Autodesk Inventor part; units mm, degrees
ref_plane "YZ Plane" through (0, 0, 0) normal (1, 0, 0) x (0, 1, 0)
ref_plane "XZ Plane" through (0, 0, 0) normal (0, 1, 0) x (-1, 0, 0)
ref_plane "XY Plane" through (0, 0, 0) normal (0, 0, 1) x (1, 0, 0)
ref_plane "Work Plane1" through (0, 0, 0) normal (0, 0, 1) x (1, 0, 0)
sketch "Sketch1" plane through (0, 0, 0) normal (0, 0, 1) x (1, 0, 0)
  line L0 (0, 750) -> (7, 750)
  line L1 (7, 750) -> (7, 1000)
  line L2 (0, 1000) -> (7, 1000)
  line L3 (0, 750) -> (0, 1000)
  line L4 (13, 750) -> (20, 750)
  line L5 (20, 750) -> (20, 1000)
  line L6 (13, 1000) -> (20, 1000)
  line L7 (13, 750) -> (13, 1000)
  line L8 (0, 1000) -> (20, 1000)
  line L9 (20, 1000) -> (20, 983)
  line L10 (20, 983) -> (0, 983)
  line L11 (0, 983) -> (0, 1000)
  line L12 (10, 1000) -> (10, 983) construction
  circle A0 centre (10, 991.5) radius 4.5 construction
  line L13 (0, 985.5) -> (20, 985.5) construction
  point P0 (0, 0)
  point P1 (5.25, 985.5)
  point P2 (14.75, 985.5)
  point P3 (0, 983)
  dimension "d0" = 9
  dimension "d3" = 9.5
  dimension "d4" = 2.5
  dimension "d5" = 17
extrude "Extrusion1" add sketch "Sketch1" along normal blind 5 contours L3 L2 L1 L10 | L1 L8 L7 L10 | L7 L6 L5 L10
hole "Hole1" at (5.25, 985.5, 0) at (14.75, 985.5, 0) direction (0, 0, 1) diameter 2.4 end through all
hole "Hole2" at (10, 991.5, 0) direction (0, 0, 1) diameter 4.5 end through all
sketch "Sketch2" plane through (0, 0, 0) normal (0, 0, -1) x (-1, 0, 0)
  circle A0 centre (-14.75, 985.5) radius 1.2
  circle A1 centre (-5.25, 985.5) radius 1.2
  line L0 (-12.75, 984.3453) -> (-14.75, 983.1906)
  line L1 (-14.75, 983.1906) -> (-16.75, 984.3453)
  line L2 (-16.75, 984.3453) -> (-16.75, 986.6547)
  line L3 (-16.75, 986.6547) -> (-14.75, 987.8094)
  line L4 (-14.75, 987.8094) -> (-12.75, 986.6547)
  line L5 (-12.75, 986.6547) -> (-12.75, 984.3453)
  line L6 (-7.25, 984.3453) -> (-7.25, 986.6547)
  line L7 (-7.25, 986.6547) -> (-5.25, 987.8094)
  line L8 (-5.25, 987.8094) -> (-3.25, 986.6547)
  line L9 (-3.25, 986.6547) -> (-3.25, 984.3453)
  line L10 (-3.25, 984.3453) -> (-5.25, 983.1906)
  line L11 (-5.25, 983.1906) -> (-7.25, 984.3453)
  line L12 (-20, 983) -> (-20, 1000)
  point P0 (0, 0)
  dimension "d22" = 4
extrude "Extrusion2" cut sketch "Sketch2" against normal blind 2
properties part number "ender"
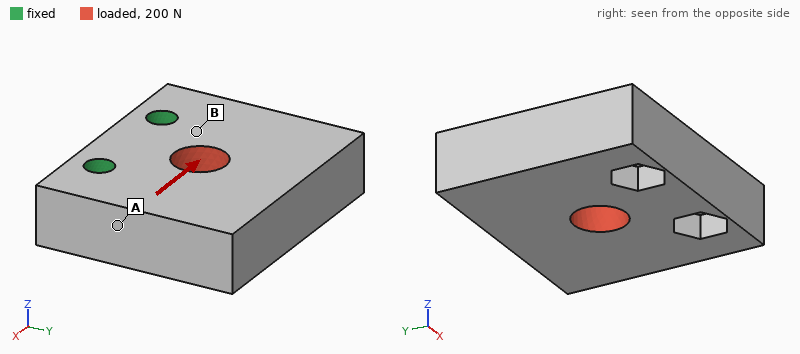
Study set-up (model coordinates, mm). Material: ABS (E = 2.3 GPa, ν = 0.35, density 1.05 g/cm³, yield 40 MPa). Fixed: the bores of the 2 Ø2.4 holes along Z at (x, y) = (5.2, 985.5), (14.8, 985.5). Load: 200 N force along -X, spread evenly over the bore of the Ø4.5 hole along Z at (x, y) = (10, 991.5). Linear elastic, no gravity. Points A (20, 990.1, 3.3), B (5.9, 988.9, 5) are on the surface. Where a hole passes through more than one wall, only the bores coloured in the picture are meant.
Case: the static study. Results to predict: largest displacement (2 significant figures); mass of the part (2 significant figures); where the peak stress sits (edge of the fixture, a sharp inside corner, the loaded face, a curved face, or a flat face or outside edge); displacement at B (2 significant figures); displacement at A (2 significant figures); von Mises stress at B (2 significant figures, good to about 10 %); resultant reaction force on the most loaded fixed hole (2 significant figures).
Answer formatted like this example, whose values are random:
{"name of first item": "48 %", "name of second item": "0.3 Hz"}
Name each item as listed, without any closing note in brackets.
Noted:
{"largest displacement": "63 µm", "mass of the part": "1.6 g", "where the peak stress sits": "edge of the fixture", "displacement at B": "16 µm", "displacement at A": "35 µm", "von Mises stress at B": "6.0 MPa", "resultant reaction force on the most loaded fixed hole": "140 N"}
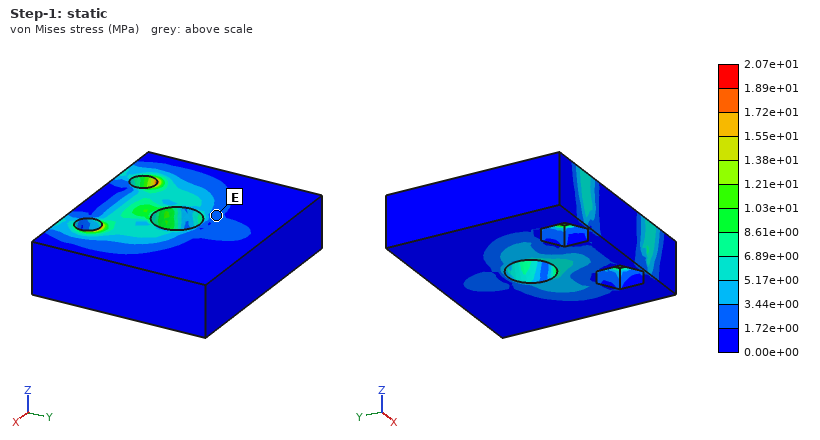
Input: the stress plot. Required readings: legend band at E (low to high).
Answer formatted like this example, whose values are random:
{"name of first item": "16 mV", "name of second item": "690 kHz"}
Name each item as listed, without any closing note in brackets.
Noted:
{"legend band at E": "1.72e+00 to 3.44e+00 MPa"}
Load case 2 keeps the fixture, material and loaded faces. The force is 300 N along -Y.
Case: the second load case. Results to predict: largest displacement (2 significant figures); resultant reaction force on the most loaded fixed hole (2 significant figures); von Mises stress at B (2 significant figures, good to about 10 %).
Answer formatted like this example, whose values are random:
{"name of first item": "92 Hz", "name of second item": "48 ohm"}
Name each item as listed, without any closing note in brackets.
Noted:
{"largest displacement": "81 µm", "resultant reaction force on the most loaded fixed hole": "150 N", "von Mises stress at B": "5.5 MPa"}
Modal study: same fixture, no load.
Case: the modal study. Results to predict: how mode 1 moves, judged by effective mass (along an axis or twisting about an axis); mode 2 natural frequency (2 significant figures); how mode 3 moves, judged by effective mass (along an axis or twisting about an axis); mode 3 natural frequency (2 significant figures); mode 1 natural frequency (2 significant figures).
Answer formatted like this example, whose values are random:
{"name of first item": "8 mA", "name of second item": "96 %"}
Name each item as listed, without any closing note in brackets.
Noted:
{"how mode 1 moves, judged by effective mass": "along Z", "mode 2 natural frequency": "6500 Hz", "how mode 3 moves, judged by effective mass": "along X", "mode 3 natural frequency": "7700 Hz", "mode 1 natural frequency": "3400 Hz"}
